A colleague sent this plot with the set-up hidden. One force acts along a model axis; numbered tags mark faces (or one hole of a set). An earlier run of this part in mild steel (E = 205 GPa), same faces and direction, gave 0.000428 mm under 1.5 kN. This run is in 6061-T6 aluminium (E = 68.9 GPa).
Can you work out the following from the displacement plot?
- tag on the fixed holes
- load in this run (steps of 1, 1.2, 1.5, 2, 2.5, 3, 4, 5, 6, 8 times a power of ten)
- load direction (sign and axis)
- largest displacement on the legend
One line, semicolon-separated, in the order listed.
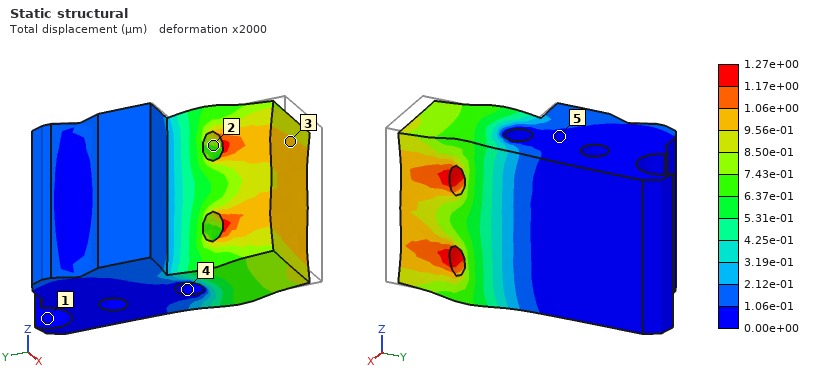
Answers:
4; 1.5 kN; +Y; 1.27e+00 µm
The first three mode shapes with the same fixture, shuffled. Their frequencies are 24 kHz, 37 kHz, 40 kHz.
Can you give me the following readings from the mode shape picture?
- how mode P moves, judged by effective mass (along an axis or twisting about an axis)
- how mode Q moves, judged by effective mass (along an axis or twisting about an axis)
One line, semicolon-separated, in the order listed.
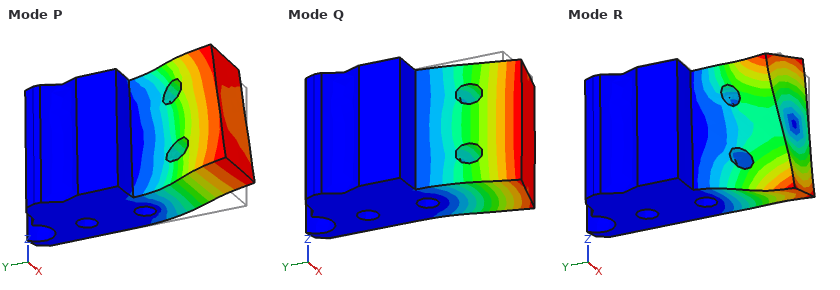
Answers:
along Z; along X
